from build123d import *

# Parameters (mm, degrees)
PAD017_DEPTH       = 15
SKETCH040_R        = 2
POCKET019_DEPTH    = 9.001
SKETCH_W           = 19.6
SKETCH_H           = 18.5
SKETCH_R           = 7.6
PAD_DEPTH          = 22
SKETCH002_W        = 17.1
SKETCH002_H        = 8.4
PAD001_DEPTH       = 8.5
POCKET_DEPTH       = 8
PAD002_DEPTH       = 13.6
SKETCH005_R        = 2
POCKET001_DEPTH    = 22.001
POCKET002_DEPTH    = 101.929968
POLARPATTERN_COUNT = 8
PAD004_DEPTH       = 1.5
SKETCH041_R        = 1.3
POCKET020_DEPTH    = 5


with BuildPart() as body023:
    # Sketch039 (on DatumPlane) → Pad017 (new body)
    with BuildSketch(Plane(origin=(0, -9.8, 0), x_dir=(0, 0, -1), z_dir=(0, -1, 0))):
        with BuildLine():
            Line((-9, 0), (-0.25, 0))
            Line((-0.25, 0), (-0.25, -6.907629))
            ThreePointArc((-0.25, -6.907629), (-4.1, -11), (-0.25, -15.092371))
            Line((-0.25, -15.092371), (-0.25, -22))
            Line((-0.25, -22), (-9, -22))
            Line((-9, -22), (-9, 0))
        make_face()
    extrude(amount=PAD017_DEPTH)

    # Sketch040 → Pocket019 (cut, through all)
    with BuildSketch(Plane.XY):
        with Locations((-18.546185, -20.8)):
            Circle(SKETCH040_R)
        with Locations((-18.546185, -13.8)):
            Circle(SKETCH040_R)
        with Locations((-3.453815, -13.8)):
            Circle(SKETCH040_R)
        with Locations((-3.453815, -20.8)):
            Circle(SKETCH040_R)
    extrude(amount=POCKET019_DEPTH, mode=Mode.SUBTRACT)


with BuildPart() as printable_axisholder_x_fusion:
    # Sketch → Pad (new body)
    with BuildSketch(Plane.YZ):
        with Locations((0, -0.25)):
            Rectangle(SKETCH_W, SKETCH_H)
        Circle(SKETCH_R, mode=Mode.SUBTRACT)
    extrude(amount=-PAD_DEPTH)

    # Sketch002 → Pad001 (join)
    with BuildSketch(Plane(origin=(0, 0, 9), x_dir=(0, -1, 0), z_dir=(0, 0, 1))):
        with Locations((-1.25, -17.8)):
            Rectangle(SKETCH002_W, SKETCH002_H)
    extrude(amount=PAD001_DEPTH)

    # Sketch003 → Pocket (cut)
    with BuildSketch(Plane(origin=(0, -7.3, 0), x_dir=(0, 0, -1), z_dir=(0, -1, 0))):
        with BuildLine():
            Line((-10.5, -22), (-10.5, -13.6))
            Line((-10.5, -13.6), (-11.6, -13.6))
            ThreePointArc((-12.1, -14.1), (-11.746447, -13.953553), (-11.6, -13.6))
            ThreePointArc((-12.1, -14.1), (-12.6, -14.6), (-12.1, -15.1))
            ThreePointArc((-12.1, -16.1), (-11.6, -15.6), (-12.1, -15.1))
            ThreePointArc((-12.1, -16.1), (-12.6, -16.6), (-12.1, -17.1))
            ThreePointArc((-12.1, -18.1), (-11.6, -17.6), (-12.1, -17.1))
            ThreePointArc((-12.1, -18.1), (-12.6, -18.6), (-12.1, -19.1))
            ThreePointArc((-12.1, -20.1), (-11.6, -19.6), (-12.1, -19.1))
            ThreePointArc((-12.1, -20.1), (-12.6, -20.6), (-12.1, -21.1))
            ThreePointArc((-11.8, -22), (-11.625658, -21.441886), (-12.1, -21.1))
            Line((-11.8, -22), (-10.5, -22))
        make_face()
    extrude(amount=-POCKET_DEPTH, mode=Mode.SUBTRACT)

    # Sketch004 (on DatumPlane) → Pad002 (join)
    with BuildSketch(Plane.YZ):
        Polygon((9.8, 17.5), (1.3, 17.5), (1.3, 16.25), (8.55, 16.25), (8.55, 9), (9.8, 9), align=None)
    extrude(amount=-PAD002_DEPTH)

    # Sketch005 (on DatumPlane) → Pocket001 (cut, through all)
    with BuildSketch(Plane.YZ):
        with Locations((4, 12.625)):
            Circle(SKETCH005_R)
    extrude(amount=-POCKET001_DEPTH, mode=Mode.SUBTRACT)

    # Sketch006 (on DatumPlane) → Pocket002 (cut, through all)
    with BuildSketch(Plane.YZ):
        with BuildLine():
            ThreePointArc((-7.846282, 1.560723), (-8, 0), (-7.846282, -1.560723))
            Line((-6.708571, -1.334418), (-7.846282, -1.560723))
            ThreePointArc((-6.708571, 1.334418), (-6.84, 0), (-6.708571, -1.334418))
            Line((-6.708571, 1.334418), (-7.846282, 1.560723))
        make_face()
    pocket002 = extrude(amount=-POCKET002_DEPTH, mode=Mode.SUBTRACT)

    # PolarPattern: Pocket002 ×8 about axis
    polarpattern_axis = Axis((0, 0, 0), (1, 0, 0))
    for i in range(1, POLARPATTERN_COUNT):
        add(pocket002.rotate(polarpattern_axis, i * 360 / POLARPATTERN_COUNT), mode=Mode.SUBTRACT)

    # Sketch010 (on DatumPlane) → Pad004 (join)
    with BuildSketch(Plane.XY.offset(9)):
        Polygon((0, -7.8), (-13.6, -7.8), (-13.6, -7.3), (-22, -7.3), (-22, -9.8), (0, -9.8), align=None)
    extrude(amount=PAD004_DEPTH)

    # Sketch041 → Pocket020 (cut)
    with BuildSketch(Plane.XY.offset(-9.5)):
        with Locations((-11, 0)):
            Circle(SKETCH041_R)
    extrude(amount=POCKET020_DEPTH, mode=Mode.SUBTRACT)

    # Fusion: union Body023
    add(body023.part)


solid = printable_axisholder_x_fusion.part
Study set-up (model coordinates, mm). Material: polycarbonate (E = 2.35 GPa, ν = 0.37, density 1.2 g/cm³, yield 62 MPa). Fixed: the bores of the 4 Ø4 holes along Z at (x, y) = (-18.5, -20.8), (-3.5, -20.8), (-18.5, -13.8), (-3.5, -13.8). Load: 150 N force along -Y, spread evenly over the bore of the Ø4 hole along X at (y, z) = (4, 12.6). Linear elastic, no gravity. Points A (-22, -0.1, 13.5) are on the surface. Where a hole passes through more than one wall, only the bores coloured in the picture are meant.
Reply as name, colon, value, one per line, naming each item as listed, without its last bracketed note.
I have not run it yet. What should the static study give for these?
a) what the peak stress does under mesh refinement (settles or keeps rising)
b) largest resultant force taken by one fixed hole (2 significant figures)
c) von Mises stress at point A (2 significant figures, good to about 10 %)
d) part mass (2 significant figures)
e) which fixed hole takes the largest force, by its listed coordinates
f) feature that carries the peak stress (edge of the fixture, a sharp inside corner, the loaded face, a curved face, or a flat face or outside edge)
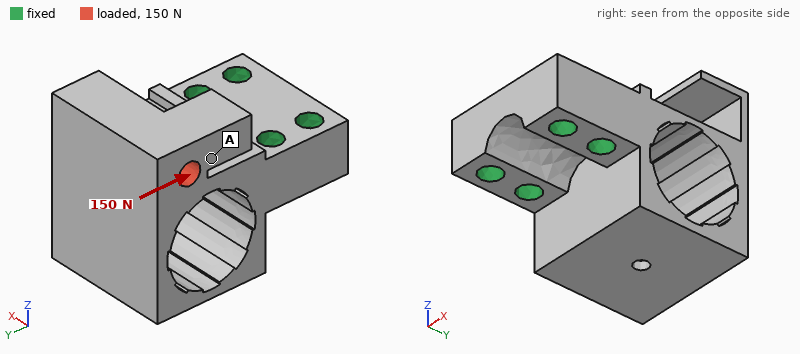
what the peak stress does under mesh refinement: keeps rising
largest resultant force taken by one fixed hole: 120 N
von Mises stress at point A: 2.0 MPa
part mass: 8.6 g
which fixed hole takes the largest force, by its listed coordinates: (-18.5, -13.8)
feature that carries the peak stress: a sharp inside corner
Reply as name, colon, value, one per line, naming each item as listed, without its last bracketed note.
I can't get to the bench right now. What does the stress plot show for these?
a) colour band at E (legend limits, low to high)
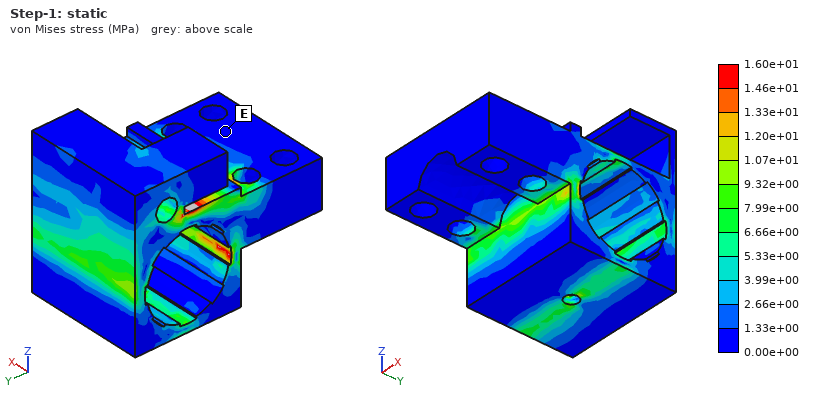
colour band at E: 0.00e+00 to 1.33e+00 MPa
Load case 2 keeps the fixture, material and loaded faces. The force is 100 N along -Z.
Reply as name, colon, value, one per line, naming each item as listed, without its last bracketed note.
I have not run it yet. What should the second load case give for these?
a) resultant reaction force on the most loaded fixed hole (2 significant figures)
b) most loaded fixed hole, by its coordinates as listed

resultant reaction force on the most loaded fixed hole: 97 N
most loaded fixed hole, by its coordinates as listed: (-18.5, -13.8)
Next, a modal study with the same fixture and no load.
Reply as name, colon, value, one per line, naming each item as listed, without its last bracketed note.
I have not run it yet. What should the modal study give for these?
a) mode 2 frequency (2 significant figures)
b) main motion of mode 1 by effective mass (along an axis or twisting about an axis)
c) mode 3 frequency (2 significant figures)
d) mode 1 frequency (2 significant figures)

mode 2 frequency: 2500 Hz
main motion of mode 1 by effective mass: along Z
mode 3 frequency: 3100 Hz
mode 1 frequency: 990 Hz
